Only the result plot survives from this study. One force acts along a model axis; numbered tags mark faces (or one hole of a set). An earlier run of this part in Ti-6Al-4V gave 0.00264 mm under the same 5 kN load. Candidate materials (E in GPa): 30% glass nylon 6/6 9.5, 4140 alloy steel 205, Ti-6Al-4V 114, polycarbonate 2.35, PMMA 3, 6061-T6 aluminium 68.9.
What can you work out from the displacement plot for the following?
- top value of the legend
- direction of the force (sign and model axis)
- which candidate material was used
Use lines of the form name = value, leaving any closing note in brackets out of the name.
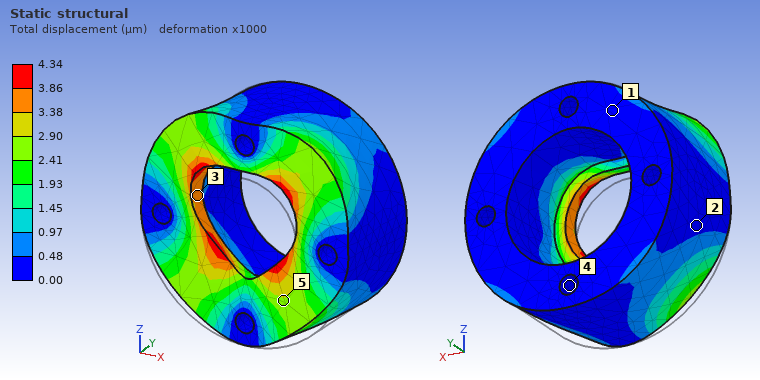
top value of the legend = 4.34 µm
direction of the force = +Z
which candidate material was used = 6061-T6 aluminium
